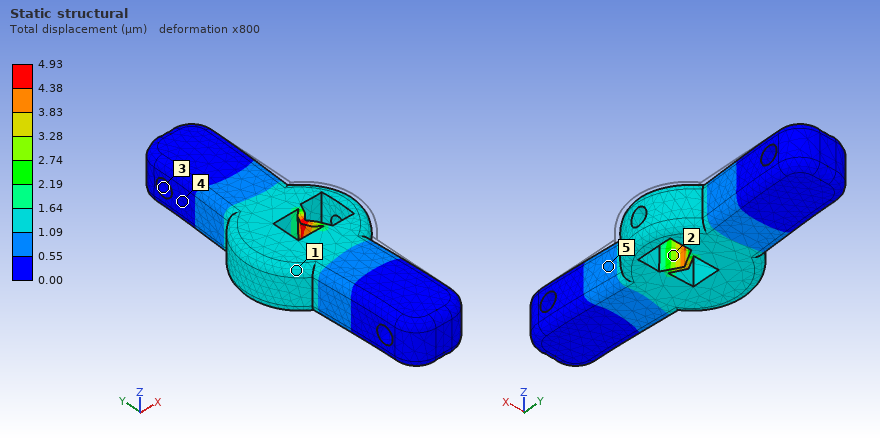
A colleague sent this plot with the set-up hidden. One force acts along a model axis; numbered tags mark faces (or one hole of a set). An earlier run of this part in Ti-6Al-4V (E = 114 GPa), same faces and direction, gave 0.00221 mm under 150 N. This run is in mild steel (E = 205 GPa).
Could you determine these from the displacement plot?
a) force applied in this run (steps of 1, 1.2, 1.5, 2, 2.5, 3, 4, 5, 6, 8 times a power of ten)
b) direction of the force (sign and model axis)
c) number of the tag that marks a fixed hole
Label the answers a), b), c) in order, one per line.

a) 600 N
b) -X
c) 3
